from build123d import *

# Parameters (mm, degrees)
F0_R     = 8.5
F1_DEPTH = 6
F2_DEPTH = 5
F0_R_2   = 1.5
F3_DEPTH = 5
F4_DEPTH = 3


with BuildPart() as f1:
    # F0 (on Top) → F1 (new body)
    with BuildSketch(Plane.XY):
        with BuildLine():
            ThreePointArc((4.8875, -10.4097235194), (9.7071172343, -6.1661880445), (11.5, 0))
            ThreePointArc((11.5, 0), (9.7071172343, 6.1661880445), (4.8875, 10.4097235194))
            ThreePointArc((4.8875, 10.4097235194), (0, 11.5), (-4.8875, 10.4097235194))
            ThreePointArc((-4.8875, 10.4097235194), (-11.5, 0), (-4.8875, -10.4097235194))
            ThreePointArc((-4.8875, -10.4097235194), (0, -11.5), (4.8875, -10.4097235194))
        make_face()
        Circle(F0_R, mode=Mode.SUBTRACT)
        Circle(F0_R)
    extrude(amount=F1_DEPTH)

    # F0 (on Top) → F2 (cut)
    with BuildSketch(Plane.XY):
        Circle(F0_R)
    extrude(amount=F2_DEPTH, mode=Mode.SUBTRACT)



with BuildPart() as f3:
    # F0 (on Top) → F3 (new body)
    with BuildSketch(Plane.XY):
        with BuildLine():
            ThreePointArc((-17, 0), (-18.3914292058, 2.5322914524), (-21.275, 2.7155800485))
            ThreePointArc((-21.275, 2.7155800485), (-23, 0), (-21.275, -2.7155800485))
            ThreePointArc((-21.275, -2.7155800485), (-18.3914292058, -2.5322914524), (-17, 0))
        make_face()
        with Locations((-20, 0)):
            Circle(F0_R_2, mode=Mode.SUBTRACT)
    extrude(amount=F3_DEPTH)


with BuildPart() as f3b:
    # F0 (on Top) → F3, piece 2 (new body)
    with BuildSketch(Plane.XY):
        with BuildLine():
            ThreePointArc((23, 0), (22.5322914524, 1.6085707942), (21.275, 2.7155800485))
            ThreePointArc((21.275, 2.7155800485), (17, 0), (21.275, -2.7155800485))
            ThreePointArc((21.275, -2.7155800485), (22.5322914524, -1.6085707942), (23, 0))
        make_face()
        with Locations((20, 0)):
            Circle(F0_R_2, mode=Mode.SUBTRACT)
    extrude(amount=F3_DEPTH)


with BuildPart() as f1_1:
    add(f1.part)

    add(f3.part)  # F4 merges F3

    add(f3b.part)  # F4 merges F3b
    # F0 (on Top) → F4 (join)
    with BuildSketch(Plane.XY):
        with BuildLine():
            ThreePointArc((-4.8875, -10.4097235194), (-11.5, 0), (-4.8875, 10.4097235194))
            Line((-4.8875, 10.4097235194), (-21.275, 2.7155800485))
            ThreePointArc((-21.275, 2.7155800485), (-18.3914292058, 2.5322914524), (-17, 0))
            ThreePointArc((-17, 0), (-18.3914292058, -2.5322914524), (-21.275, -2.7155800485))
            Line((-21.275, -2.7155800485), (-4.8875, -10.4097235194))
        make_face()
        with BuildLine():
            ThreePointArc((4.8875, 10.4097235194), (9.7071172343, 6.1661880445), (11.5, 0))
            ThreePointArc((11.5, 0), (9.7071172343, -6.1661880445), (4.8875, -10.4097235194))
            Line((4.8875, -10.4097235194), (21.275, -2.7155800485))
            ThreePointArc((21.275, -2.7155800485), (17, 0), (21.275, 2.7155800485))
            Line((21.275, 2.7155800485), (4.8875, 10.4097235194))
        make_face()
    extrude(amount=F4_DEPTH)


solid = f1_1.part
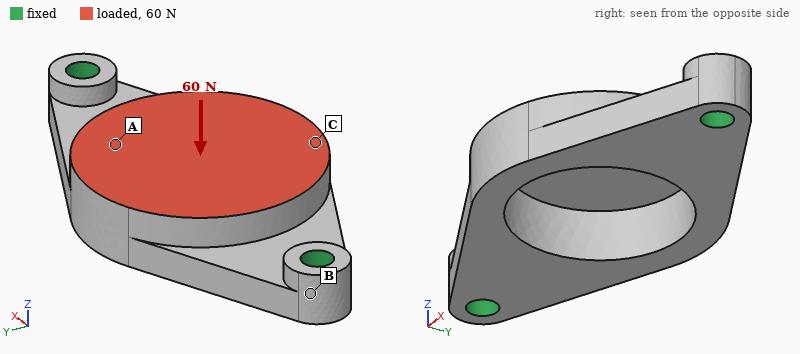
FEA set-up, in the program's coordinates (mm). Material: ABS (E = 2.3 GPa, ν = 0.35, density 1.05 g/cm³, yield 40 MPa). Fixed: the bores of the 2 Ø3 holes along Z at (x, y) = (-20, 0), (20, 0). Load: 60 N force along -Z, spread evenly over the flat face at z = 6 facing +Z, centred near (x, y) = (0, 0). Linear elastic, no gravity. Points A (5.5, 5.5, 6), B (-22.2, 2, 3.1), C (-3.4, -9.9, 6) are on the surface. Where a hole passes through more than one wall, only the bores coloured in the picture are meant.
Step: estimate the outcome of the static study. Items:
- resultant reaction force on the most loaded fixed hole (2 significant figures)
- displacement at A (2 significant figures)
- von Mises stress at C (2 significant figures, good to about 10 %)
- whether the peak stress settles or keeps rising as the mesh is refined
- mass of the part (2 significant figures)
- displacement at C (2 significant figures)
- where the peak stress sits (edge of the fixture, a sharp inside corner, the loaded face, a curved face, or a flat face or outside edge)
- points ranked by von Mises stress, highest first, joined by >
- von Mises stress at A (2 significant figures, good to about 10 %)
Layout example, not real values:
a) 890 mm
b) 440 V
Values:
a) 50 N
b) 0.090 mm
c) 2.5 MPa
d) keeps rising
e) 2.2 g
f) 0.098 mm
g) edge of the fixture
h) A > C > B
i) 5.2 MPa
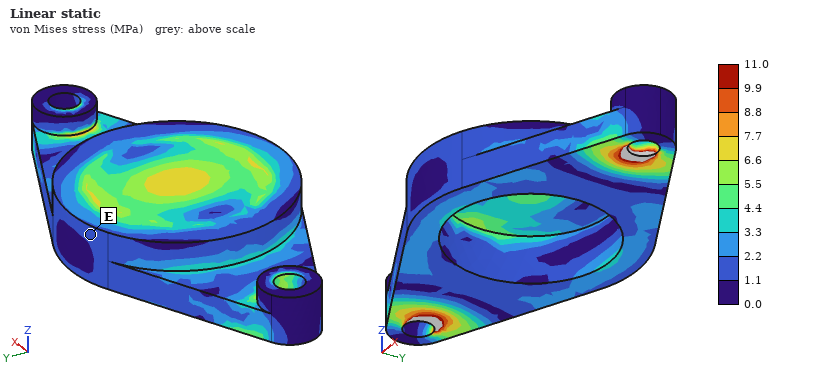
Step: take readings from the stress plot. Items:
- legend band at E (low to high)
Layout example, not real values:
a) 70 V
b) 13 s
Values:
a) 1.1 to 2.2 MPa
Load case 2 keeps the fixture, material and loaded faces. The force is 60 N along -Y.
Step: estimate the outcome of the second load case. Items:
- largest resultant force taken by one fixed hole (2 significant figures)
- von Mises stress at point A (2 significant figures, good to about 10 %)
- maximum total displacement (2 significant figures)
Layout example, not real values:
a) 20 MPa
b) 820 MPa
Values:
a) 30 N
b) 1.1 MPa
c) 0.20 mm
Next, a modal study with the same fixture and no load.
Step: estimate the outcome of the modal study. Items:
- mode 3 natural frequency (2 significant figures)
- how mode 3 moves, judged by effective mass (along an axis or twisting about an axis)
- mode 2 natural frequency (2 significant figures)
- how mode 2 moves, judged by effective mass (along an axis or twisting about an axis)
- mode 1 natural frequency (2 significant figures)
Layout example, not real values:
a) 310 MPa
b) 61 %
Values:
a) 6700 Hz
b) along Y
c) 3300 Hz
d) along Z
e) 2400 Hz
